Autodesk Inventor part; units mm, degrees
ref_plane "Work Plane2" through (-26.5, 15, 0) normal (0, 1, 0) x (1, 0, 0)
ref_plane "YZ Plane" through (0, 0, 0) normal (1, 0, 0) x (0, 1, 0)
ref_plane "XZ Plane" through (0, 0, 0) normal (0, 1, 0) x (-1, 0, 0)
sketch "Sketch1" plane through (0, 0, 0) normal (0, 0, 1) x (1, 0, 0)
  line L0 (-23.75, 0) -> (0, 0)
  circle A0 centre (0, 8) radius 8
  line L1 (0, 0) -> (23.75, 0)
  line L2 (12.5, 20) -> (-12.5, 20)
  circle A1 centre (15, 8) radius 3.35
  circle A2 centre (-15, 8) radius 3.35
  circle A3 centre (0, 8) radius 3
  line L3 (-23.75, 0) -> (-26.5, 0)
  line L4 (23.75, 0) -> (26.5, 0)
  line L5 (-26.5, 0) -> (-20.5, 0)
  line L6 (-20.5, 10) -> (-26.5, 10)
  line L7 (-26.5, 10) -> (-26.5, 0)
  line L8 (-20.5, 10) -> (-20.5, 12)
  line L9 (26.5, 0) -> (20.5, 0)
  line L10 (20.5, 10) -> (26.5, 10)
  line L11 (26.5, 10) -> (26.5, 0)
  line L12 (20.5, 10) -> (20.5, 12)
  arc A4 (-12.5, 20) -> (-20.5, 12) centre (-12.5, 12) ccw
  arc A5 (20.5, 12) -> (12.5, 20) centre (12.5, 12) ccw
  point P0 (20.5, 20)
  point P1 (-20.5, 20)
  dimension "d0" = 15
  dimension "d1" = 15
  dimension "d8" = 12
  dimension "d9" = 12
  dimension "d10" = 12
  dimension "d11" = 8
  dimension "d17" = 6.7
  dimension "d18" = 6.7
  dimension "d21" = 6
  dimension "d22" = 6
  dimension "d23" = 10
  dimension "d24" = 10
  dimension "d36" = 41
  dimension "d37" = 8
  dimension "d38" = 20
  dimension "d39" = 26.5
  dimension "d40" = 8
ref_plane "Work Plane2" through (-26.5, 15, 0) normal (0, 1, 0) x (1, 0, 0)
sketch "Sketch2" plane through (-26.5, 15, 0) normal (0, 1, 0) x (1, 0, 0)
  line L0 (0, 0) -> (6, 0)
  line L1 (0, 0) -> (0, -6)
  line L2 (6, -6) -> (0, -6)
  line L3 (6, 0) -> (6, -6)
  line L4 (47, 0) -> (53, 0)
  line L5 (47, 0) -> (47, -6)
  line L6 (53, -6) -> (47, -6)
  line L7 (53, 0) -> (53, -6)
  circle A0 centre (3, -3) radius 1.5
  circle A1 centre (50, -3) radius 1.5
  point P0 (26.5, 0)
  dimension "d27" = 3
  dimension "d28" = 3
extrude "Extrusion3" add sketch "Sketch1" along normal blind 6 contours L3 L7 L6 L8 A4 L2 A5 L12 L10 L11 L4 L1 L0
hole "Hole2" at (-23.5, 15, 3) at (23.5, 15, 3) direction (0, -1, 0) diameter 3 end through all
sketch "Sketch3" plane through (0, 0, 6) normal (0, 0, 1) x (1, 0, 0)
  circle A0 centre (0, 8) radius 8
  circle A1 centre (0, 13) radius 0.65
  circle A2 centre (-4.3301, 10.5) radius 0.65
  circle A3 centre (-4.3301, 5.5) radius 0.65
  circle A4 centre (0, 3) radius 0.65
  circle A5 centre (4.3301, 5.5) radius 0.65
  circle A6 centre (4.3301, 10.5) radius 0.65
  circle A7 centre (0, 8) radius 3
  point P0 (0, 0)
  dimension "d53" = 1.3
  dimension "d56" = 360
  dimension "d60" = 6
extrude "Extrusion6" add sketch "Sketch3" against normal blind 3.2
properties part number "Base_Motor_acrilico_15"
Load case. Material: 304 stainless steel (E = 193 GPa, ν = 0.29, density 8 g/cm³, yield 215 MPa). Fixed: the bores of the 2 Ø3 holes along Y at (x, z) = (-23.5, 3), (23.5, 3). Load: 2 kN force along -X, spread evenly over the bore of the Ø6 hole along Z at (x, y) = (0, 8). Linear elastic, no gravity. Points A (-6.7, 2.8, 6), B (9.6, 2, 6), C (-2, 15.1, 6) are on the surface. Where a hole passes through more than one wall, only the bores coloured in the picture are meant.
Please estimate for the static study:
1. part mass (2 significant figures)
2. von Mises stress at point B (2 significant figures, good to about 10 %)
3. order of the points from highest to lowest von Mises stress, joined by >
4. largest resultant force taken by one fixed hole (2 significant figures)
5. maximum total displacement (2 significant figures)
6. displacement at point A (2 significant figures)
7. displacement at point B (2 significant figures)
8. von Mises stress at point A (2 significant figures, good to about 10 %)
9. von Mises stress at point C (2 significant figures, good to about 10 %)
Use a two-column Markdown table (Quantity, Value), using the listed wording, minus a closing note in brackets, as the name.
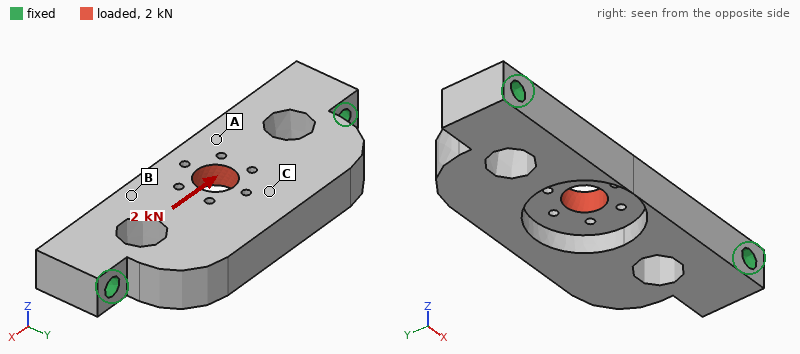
| Quantity | Value |
|---|---|
| part mass | 34 g |
| von Mises stress at point B | 28 MPa |
| order of the points from highest to lowest von Mises stress, joined by > | B > A > C |
| largest resultant force taken by one fixed hole | 1.0 kN |
| maximum total displacement | 3.7 µm |
| displacement at point A | 2.0 µm |
| displacement at point B | 1.6 µm |
| von Mises stress at point A | 22 MPa |
| von Mises stress at point C | 5.6 MPa |
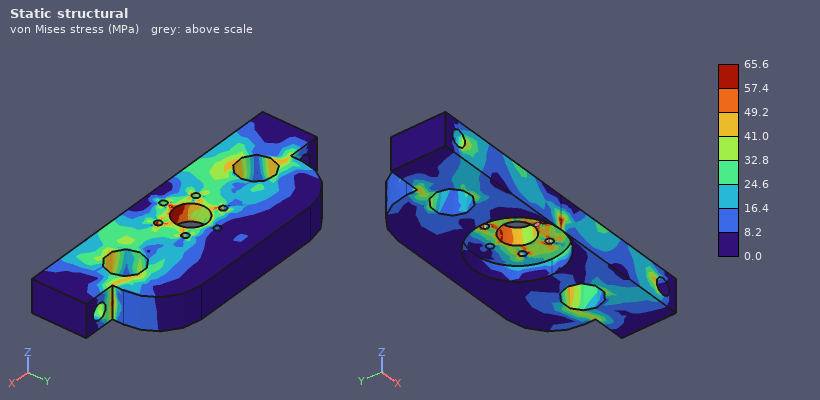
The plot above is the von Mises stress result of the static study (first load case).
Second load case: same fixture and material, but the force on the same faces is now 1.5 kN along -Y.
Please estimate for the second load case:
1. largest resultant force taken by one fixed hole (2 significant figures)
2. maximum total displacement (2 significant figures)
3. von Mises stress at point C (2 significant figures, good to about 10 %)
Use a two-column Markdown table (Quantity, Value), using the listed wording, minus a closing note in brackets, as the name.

| Quantity | Value |
|---|---|
| largest resultant force taken by one fixed hole | 930 N |
| maximum total displacement | 8.7 µm |
| von Mises stress at point C | 25 MPa |
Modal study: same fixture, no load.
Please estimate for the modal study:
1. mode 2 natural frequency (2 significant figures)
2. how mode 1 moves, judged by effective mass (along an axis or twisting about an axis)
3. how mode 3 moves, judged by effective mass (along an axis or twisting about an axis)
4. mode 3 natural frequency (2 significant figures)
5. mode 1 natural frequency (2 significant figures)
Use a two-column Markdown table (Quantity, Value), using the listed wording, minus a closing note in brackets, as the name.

| Quantity | Value |
|---|---|
| mode 2 natural frequency | 14 kHz |
| how mode 1 moves, judged by effective mass | along Z |
| how mode 3 moves, judged by effective mass | twisting about Y |
| mode 3 natural frequency | 19 kHz |
| mode 1 natural frequency | 7800 Hz |
